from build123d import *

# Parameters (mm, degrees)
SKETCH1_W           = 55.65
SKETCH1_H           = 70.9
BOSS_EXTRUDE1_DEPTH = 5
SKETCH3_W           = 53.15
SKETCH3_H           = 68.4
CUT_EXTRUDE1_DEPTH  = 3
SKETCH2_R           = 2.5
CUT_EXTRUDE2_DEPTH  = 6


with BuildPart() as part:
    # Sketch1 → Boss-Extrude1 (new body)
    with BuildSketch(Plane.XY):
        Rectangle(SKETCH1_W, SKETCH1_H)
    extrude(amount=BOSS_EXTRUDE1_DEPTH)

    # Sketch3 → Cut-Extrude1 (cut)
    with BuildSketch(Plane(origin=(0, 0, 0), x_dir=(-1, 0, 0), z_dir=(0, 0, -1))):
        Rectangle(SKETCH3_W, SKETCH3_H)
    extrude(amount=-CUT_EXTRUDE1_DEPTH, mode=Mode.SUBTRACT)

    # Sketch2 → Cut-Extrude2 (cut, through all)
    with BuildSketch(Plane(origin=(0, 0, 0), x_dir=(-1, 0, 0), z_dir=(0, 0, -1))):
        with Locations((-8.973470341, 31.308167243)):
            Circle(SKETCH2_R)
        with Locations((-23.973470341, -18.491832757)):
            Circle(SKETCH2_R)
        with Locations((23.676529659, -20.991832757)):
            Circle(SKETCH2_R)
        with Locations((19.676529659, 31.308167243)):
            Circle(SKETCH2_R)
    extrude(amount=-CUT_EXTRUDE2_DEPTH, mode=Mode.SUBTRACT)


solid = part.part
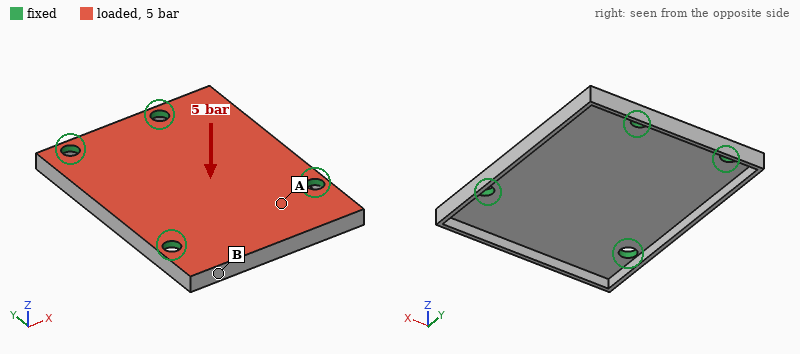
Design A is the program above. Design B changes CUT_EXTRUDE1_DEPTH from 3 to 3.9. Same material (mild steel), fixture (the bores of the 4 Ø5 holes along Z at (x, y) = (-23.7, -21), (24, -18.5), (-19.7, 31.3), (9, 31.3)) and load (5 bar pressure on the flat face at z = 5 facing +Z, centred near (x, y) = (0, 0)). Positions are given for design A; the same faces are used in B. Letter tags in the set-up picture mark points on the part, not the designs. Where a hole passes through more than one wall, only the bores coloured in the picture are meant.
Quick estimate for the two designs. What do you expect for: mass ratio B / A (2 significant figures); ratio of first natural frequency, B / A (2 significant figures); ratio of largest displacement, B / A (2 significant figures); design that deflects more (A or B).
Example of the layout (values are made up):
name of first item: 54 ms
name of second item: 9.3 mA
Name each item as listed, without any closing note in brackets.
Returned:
mass ratio B / A: 0.63
ratio of first natural frequency, B / A: 0.61
ratio of largest displacement, B / A: 5.3
design that deflects more: B
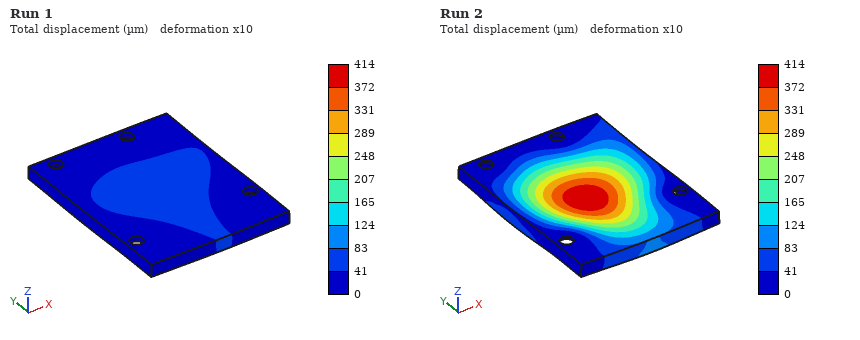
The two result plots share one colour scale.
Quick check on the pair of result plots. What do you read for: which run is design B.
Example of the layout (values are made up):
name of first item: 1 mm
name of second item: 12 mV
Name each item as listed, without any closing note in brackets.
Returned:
which run is design B: Run 2
